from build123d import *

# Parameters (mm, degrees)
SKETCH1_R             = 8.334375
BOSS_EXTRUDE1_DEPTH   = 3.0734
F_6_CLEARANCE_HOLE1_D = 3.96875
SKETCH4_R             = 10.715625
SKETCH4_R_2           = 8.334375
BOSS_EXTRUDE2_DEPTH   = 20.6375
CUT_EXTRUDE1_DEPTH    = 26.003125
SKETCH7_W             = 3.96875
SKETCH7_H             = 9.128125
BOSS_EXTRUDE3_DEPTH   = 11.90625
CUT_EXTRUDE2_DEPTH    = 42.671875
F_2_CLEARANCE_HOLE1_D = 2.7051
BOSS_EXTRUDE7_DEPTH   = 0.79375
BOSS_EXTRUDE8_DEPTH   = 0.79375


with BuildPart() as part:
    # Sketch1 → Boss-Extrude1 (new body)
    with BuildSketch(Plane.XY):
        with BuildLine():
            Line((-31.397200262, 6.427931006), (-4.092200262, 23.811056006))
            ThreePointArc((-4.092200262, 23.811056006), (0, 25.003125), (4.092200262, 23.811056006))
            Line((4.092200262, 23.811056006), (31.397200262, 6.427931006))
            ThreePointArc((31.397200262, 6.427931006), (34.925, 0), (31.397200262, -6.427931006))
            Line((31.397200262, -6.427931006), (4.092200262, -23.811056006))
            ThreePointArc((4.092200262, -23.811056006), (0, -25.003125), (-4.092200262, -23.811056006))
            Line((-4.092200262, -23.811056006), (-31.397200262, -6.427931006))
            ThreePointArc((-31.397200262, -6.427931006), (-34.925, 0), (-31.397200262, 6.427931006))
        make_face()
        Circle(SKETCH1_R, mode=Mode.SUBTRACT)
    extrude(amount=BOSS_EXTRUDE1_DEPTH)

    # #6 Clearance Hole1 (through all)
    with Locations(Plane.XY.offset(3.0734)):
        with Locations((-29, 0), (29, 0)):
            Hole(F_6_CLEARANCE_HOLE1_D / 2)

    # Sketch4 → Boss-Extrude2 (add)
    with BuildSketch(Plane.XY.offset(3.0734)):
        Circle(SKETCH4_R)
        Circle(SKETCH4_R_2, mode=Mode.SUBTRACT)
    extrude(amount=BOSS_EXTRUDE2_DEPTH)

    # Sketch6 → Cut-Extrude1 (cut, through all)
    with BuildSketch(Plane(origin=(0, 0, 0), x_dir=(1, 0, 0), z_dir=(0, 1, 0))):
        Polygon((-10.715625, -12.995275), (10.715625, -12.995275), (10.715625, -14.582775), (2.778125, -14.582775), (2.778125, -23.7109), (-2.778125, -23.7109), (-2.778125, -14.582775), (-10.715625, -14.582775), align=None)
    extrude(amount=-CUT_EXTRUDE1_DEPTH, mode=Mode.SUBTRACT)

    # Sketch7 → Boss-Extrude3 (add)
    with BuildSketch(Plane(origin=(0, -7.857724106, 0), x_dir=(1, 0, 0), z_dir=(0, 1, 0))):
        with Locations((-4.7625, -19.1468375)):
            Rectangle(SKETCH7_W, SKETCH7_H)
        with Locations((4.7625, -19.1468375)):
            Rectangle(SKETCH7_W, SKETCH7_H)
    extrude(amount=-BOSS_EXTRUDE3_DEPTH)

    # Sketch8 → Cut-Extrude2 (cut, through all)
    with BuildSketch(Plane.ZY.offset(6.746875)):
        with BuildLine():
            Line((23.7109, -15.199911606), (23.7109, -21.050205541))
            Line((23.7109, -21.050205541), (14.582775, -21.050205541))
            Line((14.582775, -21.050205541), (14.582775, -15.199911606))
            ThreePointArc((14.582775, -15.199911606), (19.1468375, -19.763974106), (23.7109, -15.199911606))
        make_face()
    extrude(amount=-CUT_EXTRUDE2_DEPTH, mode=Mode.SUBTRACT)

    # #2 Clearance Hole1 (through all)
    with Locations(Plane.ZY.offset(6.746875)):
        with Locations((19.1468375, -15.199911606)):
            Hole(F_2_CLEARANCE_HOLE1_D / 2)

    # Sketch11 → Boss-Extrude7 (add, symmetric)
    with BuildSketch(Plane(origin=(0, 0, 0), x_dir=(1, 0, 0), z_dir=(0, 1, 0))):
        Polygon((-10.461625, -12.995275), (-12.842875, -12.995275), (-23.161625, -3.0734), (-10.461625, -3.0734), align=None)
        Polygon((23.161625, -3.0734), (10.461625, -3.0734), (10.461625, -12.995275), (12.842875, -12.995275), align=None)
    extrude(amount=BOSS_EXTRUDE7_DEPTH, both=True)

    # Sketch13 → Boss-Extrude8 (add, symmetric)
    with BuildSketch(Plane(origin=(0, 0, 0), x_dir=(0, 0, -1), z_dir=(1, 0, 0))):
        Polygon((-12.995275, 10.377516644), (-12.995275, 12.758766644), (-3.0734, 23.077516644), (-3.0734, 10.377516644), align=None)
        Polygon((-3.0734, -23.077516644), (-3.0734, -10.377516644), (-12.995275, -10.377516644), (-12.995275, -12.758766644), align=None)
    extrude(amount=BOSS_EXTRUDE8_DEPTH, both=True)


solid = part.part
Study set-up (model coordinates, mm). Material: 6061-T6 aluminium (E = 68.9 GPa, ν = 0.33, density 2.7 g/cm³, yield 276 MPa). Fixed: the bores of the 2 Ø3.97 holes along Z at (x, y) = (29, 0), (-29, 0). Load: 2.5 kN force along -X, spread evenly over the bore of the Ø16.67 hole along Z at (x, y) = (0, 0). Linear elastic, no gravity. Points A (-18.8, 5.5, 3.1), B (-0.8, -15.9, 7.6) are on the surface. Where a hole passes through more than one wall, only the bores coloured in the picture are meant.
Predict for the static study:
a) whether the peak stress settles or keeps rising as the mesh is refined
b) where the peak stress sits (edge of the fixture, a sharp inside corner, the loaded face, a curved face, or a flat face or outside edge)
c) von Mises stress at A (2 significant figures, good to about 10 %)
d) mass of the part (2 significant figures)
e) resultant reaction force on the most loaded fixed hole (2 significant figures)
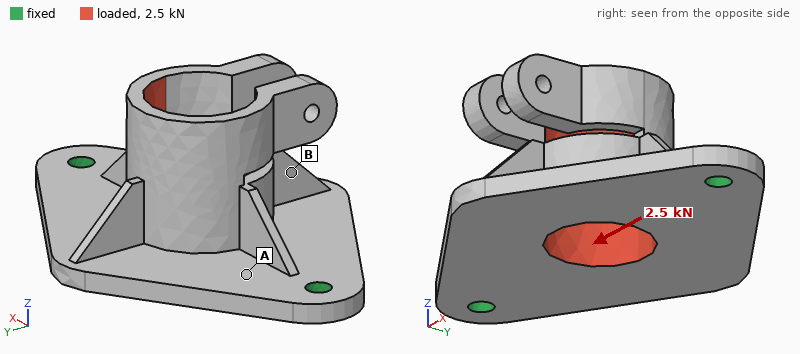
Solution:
keeps rising
a sharp inside corner
40 MPa
26 g
1.4 kN
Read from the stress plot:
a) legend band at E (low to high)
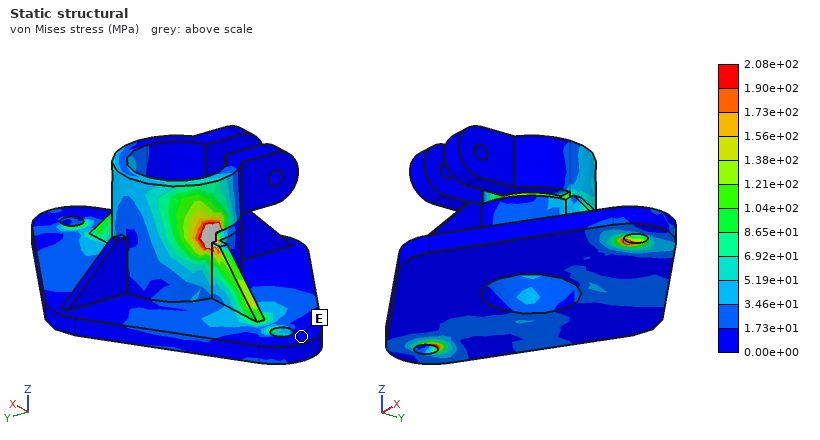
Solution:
0.00e+00 to 1.73e+01 MPa
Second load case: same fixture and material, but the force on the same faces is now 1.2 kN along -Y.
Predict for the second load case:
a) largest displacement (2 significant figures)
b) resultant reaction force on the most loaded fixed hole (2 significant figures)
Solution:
0.53 mm
610 N
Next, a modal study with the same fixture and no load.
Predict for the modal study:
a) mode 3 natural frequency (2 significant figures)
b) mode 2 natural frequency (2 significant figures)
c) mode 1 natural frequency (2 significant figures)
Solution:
2500 Hz
2300 Hz
1900 Hz
